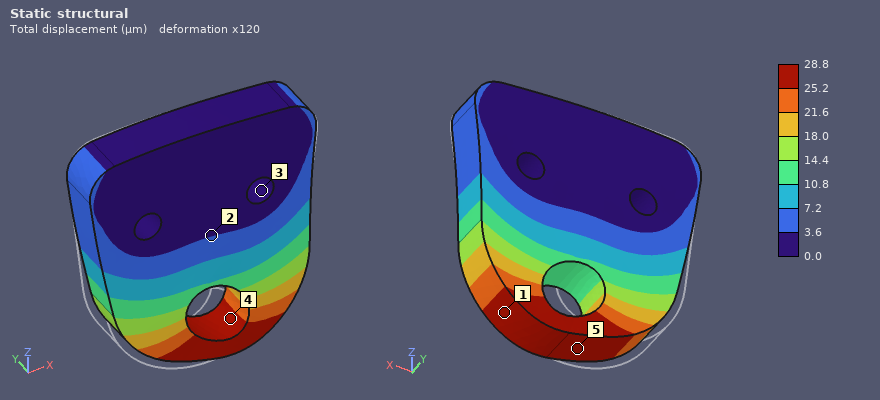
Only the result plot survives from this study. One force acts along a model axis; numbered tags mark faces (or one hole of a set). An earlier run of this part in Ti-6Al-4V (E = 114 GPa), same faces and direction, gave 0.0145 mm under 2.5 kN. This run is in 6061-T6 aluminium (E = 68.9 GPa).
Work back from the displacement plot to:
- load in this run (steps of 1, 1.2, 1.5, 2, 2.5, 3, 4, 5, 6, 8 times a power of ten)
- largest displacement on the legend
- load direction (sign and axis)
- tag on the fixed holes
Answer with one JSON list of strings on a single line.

["3 kN", "28.8 µm", "+X", "3"]
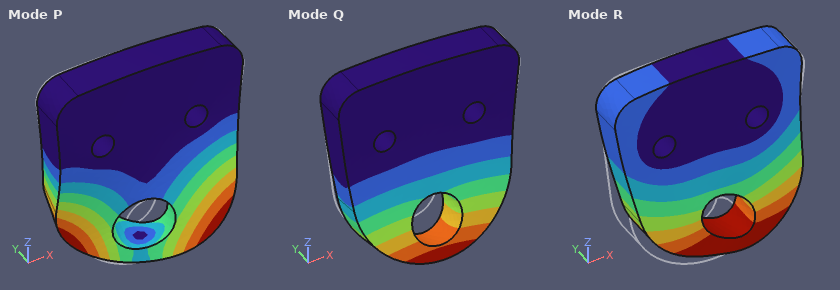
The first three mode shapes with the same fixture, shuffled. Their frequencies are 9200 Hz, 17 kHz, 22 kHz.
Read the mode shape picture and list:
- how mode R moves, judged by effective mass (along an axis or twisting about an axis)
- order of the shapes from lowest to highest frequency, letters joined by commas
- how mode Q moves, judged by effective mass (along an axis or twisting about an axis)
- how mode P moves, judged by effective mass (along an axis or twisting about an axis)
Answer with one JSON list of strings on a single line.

["along X", "Q, P, R", "along Y", "twisting about Z"]
